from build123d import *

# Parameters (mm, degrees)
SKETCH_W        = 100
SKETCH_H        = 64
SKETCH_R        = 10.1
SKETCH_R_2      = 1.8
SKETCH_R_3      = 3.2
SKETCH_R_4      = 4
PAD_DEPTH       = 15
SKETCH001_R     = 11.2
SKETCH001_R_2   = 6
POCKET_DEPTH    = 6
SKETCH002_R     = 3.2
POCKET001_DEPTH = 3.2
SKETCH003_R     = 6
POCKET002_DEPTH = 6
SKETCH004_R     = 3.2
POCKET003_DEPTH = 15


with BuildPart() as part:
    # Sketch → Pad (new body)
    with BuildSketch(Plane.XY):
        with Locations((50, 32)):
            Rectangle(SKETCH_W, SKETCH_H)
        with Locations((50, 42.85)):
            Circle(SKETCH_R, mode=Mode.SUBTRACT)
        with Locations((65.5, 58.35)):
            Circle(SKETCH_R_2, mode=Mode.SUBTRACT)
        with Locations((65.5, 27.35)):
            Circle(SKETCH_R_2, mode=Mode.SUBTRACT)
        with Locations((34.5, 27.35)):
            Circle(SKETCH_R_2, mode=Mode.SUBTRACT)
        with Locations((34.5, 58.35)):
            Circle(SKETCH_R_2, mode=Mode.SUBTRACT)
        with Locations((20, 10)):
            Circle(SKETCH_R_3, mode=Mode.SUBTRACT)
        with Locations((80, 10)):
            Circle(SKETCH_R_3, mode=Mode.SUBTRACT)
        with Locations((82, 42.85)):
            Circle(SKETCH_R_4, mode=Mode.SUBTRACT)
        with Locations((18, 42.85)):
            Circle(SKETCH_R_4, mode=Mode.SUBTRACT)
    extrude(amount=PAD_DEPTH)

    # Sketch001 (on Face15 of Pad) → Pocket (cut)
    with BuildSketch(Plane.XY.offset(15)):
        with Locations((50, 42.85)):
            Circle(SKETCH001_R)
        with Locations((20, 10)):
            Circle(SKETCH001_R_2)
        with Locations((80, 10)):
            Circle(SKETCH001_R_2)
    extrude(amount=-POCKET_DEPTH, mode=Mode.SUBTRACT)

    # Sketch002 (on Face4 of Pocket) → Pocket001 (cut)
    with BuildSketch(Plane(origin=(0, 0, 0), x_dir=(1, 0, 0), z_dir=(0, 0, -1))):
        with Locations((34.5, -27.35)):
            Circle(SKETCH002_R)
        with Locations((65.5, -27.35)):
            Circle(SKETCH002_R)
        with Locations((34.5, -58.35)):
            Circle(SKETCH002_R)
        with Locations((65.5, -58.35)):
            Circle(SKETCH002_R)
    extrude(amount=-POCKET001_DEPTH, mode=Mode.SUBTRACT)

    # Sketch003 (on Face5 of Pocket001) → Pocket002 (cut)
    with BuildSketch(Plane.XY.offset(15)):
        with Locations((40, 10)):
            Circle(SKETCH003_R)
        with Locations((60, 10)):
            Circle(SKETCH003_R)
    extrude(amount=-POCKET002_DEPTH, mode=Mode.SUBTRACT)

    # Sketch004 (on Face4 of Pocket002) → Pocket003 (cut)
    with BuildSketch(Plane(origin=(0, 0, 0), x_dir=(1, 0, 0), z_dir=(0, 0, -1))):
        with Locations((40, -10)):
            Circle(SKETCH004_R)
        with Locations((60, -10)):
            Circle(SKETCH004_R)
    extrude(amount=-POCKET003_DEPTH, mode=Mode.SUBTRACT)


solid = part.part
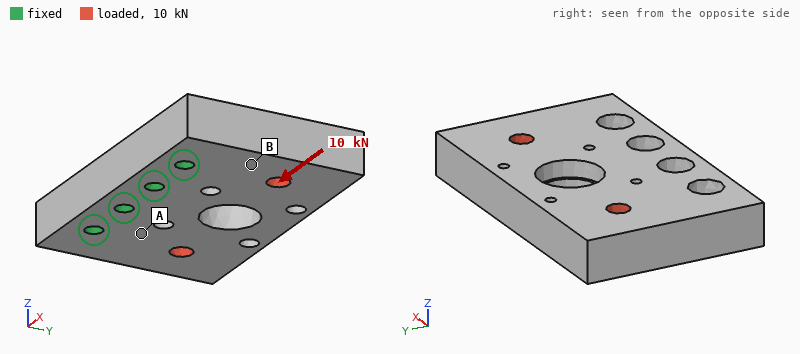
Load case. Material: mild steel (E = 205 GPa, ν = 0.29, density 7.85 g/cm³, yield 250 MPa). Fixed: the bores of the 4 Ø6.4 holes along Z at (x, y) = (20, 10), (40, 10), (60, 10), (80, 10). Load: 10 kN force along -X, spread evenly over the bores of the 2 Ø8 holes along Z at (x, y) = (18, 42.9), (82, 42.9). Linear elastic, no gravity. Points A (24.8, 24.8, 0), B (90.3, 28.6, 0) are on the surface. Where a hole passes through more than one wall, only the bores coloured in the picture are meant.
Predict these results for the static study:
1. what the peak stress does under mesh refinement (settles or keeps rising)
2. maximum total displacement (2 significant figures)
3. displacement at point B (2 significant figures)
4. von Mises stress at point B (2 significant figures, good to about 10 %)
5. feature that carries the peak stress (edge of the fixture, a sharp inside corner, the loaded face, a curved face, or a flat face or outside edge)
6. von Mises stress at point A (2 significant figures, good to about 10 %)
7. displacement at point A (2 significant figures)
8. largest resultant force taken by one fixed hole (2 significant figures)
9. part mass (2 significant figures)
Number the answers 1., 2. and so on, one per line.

1. keeps rising
2. 11 µm
3. 5.1 µm
4. 9.8 MPa
5. edge of the fixture
6. 24 MPa
7. 2.9 µm
8. 5.4 kN
9. 660 g
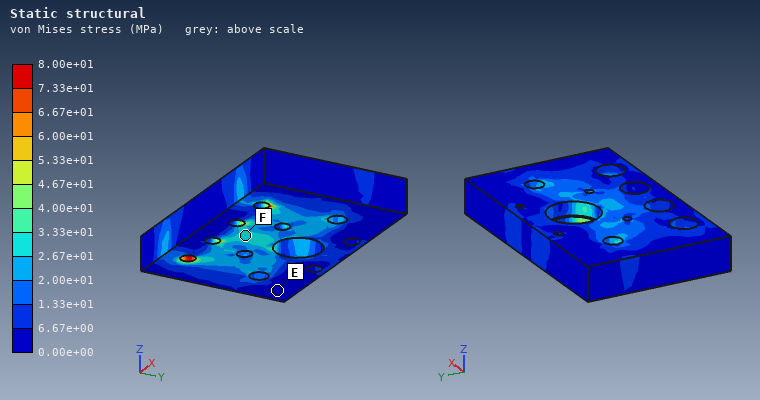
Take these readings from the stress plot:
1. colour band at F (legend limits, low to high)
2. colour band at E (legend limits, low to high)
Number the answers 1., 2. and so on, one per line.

1. 2.67e+01 to 3.33e+01 MPa
2. 0.00e+00 to 6.67e+00 MPa
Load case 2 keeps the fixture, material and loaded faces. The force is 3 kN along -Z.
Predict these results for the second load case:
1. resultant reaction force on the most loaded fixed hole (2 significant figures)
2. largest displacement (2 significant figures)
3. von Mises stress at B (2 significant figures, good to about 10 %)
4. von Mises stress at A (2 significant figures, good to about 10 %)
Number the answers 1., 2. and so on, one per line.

1. 1.0 kN
2. 29 µm
3. 11 MPa
4. 17 MPa
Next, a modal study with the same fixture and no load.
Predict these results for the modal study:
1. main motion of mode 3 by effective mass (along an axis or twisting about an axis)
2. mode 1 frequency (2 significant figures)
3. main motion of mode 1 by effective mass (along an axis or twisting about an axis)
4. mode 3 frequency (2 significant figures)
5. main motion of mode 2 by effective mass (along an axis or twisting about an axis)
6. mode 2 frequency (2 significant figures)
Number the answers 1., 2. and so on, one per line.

1. along X
2. 2900 Hz
3. along Z
4. 8200 Hz
5. twisting about Y
6. 4400 Hz
